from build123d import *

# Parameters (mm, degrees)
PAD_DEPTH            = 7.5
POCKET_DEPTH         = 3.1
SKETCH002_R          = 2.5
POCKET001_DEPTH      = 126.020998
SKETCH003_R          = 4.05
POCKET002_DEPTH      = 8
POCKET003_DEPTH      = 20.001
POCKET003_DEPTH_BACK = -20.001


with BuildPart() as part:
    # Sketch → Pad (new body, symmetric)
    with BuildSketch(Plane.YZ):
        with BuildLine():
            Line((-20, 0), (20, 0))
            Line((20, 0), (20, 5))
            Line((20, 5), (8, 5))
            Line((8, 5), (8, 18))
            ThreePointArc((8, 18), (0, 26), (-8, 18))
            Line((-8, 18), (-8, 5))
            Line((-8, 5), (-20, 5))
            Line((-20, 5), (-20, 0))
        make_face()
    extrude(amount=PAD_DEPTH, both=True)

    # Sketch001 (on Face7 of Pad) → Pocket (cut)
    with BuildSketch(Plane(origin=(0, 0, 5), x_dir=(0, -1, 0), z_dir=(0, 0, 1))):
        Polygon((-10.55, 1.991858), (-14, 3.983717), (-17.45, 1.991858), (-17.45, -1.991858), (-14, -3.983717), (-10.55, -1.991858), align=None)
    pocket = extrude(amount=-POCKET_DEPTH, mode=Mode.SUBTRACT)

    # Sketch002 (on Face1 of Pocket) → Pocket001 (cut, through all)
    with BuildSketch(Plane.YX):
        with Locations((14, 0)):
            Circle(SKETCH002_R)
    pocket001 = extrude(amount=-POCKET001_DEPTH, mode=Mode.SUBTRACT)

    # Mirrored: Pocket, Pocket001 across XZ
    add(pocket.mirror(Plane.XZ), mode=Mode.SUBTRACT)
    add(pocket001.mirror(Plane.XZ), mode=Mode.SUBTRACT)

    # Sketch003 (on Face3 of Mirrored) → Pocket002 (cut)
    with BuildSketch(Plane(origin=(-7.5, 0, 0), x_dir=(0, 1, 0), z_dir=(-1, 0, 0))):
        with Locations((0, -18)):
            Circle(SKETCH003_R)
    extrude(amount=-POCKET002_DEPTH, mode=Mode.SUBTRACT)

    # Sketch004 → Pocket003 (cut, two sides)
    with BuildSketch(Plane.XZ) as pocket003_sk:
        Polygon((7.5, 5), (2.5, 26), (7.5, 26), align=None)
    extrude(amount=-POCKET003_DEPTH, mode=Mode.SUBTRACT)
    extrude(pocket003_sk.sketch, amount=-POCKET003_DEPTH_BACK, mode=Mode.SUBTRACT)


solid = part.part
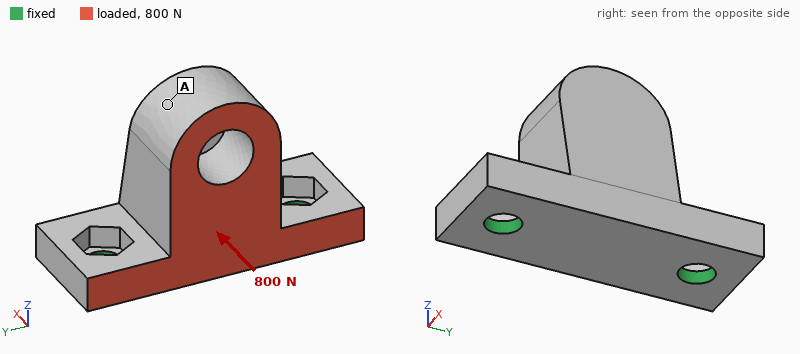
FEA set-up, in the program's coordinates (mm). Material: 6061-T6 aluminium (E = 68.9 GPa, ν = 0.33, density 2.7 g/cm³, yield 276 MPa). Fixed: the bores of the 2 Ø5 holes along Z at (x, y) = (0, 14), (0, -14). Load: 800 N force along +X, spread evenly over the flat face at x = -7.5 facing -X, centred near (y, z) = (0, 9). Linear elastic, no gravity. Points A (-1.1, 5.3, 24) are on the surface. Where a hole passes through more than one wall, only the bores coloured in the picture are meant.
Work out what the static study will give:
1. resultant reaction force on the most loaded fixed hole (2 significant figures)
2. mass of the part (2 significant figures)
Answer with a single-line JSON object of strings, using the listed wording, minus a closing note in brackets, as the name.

{"resultant reaction force on the most loaded fixed hole": "400 N", "mass of the part": "17 g"}
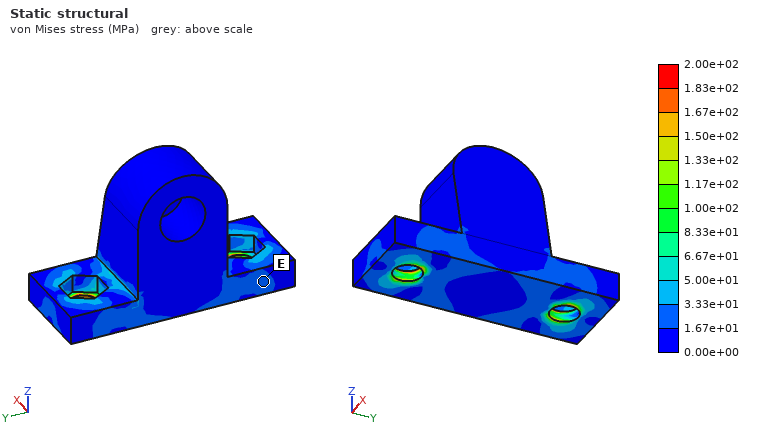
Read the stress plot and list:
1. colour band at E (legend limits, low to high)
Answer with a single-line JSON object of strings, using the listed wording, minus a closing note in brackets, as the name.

{"colour band at E": "1.67e+01 to 3.33e+01 MPa"}
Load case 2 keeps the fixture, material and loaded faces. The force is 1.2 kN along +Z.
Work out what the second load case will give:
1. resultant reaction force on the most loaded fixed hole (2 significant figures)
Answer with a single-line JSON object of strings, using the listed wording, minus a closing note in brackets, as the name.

{"resultant reaction force on the most loaded fixed hole": "690 N"}
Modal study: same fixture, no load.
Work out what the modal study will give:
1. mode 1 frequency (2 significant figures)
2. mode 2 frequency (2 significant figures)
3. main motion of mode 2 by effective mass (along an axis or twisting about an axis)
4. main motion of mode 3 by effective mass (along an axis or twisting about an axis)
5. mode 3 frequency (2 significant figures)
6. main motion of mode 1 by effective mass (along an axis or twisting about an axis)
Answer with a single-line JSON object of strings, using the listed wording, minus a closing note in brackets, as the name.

{"mode 1 frequency": "5000 Hz", "mode 2 frequency": "15 kHz", "main motion of mode 2 by effective mass": "along Y", "main motion of mode 3 by effective mass": "along Z", "mode 3 frequency": "17 kHz", "main motion of mode 1 by effective mass": "along X"}
